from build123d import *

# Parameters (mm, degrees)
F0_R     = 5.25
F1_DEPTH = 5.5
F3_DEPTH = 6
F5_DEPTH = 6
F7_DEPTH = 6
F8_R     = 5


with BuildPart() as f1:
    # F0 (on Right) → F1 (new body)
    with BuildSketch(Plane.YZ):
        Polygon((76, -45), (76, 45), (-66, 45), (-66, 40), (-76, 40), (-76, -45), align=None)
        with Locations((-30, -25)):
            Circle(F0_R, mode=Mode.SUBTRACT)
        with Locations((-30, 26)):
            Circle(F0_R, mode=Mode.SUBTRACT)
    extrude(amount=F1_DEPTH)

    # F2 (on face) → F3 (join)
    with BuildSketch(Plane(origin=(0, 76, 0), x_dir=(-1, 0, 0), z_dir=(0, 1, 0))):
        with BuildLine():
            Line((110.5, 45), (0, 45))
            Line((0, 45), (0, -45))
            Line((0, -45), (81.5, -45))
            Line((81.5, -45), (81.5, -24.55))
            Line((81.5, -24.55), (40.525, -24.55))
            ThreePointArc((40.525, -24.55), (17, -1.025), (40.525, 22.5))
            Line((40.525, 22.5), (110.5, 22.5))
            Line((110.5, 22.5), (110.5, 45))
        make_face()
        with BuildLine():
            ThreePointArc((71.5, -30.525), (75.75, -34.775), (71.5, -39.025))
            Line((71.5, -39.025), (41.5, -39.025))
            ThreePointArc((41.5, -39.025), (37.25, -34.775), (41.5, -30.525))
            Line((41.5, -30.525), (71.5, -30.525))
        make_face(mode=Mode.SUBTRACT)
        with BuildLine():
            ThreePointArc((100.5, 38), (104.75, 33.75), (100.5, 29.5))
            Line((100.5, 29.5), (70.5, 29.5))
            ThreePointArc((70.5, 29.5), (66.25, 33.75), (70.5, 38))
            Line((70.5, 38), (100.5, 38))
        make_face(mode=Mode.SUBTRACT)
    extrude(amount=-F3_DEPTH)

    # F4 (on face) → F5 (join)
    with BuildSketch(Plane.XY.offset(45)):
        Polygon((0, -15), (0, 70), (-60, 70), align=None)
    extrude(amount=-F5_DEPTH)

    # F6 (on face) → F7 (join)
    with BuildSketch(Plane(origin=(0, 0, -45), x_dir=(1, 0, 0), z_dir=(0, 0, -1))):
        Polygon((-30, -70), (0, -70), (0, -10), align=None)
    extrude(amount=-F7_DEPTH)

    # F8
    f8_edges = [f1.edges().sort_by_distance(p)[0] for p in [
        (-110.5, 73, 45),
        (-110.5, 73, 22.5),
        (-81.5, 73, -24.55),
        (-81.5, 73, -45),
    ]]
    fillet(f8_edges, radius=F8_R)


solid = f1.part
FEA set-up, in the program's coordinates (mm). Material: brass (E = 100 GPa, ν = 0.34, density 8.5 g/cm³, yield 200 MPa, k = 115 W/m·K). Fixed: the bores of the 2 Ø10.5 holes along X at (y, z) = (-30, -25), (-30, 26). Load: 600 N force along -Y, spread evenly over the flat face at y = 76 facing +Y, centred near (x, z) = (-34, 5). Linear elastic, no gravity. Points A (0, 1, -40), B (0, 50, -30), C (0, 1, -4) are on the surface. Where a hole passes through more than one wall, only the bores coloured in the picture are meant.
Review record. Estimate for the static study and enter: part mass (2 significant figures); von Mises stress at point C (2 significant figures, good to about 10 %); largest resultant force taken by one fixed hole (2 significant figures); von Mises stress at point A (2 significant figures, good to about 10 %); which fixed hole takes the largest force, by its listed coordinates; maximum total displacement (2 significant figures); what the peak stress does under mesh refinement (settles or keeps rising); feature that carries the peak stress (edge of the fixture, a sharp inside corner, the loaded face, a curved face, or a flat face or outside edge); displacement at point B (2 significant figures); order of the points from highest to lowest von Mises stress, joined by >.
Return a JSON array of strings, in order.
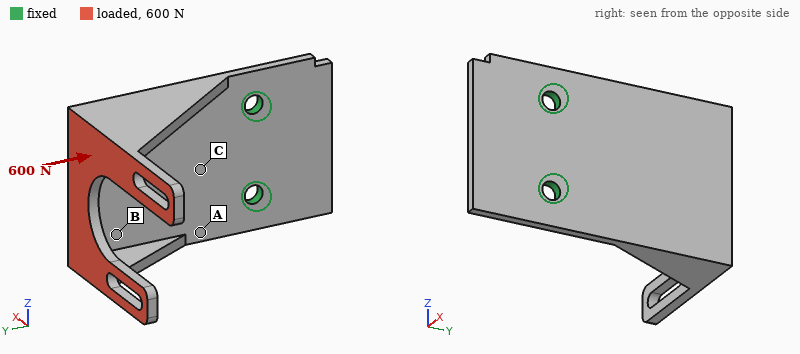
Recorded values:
["1.0 kg", "28 MPa", "350 N", "43 MPa", "(-30, 26)", "0.96 mm", "keeps rising", "edge of the fixture", "0.31 mm", "A > C > B"]
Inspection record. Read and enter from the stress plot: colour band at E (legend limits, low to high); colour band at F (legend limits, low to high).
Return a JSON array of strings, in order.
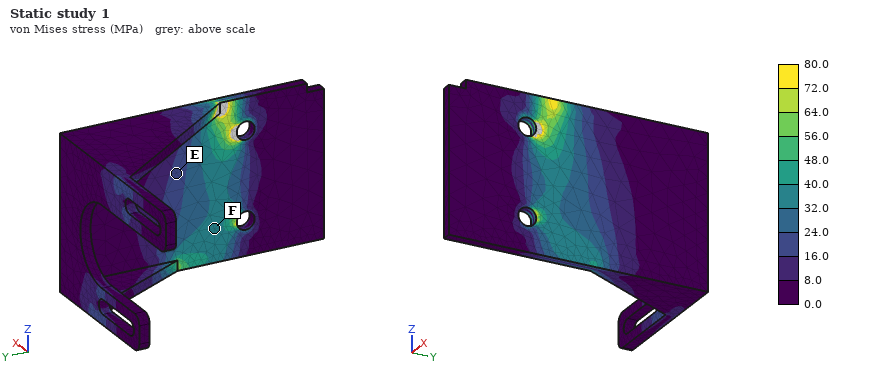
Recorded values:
["16.0 to 24.0 MPa", "32.0 to 40.0 MPa"]
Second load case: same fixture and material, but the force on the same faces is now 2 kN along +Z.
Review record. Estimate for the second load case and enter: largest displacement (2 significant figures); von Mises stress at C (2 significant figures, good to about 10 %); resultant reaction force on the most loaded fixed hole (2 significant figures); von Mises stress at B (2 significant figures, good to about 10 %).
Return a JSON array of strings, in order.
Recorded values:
["2.4 mm", "81 MPa", "4.0 kN", "65 MPa"]
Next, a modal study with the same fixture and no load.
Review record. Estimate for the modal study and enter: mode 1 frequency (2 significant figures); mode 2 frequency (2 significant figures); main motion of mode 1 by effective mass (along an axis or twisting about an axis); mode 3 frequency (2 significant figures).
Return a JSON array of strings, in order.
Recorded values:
["160 Hz", "290 Hz", "along X", "880 Hz"]
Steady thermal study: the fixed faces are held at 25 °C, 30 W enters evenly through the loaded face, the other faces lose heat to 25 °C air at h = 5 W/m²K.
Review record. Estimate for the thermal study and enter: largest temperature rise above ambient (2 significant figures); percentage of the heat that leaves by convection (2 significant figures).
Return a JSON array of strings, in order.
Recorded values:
["58 K", "16 %"]
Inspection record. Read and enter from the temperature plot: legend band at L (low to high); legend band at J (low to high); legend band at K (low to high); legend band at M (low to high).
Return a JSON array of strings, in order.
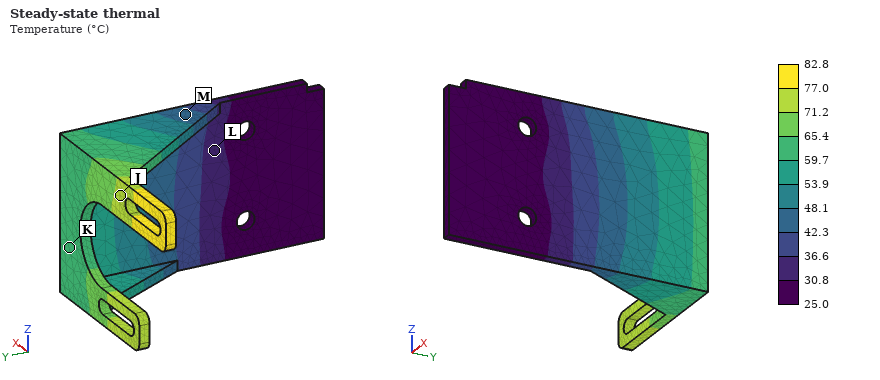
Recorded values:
["30.8 to 36.6 °C", "71.2 to 77.0 °C", "59.7 to 65.4 °C", "42.3 to 48.1 °C"]
